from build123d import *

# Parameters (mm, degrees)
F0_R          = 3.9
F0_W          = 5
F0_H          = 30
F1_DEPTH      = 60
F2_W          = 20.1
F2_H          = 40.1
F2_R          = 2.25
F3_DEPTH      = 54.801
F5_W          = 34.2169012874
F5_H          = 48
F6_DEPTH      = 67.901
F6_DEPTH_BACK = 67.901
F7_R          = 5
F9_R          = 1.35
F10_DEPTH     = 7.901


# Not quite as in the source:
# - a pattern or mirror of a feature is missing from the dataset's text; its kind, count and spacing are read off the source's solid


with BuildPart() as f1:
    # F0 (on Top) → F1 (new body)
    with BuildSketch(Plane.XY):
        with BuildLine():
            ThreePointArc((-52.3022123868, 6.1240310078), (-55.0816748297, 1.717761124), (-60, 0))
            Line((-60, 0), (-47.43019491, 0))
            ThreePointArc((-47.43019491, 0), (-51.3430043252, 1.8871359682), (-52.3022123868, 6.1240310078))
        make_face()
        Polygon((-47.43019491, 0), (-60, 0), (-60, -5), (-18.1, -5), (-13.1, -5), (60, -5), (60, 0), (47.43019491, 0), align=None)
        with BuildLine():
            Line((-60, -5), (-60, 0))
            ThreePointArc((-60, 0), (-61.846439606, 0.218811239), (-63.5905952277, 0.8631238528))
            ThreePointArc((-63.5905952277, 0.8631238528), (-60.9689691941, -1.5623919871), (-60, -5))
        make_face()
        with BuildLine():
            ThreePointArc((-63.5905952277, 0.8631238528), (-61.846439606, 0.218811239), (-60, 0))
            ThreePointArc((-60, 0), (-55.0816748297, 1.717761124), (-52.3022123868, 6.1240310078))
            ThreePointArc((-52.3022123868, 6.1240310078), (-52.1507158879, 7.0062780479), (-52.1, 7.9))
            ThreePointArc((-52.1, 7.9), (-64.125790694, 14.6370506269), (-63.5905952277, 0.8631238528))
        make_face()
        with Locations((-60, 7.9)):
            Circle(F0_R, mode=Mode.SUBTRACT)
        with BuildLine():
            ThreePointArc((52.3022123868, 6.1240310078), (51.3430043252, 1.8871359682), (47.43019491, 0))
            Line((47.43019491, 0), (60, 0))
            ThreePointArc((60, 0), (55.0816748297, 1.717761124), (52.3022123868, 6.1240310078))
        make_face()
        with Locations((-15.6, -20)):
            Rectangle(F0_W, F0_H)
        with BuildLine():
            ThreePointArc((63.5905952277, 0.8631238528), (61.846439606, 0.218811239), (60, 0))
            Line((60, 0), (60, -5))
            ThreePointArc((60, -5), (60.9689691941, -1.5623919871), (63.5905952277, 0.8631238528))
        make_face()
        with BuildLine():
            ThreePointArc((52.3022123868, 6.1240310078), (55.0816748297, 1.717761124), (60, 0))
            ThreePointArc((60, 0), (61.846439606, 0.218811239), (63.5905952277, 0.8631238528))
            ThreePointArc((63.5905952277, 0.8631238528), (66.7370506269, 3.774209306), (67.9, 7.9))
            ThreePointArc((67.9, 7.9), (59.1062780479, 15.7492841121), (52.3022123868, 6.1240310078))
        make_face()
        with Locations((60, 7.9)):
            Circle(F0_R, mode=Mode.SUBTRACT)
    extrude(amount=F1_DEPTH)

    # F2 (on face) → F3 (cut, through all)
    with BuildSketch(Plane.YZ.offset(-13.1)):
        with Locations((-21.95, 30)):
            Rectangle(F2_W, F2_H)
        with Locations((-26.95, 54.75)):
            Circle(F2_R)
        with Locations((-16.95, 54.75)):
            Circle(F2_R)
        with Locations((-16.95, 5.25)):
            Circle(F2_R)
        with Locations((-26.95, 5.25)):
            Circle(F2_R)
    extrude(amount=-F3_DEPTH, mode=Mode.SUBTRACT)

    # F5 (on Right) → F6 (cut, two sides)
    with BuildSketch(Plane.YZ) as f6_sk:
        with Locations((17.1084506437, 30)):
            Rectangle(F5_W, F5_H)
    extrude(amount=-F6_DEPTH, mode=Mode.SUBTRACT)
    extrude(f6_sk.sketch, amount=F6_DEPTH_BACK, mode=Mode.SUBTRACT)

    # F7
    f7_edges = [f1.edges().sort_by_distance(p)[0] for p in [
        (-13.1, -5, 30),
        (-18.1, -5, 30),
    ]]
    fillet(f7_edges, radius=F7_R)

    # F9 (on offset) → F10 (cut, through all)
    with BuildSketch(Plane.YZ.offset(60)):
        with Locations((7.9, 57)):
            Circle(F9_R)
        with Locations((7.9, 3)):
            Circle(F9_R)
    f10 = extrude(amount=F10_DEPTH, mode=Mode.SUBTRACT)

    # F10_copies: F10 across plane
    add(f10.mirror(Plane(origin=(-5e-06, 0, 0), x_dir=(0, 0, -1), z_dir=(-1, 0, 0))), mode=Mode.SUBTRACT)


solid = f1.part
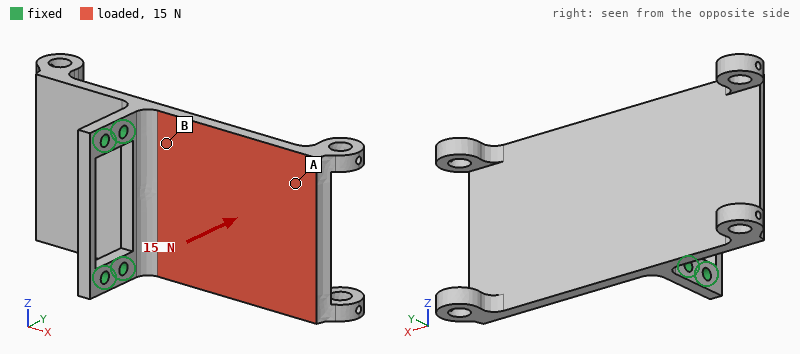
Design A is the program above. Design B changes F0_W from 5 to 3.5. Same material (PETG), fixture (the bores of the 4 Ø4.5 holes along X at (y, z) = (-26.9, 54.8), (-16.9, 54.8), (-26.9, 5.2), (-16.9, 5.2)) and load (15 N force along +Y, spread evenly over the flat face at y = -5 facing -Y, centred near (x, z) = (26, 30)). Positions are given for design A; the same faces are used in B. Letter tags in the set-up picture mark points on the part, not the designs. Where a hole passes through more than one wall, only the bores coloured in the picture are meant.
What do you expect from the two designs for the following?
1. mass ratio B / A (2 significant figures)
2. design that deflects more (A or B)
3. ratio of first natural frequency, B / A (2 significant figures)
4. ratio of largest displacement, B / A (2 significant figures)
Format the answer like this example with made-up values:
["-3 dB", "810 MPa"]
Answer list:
["0.97", "B", "0.69", "2.0"]
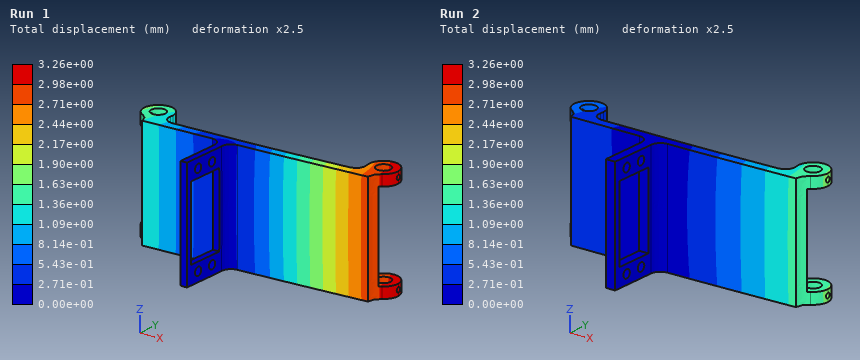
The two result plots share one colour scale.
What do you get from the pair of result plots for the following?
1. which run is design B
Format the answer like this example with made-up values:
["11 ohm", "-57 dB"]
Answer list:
["Run 1"]
